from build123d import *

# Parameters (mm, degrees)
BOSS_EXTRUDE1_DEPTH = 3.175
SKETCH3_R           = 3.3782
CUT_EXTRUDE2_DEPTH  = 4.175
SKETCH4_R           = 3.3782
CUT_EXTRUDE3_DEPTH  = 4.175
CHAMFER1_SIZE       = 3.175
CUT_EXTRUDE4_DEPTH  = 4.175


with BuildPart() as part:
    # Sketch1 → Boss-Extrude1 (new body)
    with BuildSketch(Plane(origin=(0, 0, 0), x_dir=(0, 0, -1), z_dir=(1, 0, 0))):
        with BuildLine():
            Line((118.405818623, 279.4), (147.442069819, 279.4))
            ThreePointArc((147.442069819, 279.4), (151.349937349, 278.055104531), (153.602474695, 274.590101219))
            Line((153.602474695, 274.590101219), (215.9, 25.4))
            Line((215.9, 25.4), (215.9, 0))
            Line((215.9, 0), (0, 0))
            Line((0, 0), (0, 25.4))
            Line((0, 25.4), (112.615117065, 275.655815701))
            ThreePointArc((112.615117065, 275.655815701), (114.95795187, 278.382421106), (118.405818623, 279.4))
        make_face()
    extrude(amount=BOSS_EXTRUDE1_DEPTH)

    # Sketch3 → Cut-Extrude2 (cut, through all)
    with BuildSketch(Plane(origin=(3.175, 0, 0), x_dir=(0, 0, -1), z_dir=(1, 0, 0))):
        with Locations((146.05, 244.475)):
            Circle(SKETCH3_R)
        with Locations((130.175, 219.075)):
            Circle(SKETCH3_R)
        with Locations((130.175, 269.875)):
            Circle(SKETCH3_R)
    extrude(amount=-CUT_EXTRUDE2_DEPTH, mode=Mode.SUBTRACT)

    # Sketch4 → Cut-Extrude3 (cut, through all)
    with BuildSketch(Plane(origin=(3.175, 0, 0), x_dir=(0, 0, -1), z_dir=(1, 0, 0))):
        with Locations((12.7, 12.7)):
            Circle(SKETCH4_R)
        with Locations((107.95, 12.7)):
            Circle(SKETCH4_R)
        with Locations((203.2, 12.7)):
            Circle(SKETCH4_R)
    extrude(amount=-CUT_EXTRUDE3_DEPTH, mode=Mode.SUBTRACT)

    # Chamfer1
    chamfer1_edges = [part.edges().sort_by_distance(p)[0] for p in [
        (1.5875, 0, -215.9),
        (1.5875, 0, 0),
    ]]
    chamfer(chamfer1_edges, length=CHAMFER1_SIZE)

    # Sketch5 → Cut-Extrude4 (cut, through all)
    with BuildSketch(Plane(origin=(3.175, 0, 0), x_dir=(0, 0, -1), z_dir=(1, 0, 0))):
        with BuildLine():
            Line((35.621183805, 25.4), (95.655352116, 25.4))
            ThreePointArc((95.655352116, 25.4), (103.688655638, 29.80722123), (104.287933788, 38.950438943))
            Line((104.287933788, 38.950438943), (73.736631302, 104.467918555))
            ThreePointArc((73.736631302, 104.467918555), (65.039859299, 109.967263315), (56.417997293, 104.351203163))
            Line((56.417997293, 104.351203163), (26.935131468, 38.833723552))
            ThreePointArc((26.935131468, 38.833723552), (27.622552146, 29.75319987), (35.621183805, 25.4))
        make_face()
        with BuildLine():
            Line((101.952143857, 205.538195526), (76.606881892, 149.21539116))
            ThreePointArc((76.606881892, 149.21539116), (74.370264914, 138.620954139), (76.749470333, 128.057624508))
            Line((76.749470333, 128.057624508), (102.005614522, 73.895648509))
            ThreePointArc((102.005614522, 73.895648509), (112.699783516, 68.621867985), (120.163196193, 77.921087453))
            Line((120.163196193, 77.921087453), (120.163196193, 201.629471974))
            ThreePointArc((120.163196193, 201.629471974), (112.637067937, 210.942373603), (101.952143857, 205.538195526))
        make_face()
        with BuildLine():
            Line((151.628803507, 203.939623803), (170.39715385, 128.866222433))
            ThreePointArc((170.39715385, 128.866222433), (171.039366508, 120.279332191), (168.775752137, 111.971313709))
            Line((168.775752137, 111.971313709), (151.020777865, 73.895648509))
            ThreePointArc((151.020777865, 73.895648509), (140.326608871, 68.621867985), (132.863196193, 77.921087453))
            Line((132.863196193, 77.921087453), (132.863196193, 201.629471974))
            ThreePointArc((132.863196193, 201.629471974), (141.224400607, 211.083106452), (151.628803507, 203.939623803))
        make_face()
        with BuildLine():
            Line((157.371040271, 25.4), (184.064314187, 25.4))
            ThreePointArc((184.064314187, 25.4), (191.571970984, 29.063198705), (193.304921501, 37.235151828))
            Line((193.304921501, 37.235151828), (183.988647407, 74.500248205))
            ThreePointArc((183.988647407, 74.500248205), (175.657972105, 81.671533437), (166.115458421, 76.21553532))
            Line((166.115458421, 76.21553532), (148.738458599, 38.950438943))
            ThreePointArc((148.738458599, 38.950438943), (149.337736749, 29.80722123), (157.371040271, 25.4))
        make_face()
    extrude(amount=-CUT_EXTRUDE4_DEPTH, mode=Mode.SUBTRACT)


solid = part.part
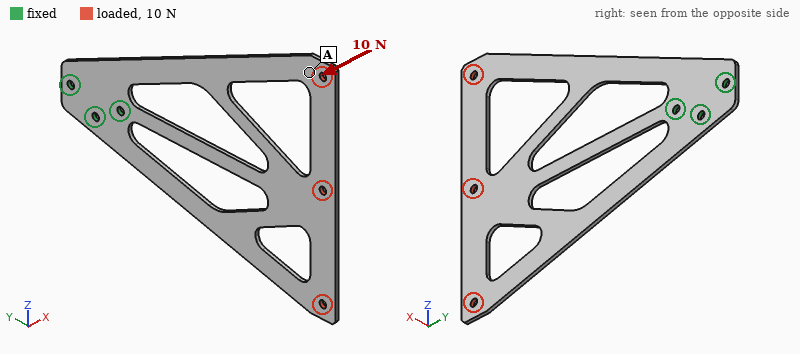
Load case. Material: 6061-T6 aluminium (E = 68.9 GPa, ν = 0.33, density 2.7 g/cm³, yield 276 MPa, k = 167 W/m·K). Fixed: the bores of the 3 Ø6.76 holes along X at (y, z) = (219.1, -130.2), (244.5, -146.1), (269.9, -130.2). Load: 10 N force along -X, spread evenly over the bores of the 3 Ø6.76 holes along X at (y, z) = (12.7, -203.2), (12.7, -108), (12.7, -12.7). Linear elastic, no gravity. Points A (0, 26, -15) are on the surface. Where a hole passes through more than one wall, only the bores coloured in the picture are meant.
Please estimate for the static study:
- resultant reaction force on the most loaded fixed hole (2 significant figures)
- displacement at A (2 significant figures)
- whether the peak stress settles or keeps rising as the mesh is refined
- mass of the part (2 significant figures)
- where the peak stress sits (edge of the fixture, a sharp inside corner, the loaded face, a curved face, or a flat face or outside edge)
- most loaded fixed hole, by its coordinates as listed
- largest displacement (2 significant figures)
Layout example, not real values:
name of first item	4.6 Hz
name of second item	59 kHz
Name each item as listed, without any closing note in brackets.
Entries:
resultant reaction force on the most loaded fixed hole	46 N
displacement at A	3.2 mm
whether the peak stress settles or keeps rising as the mesh is refined	keeps rising
mass of the part	200 g
where the peak stress sits	edge of the fixture
most loaded fixed hole, by its coordinates as listed	(219.1, -130.2)
largest displacement	3.8 mm
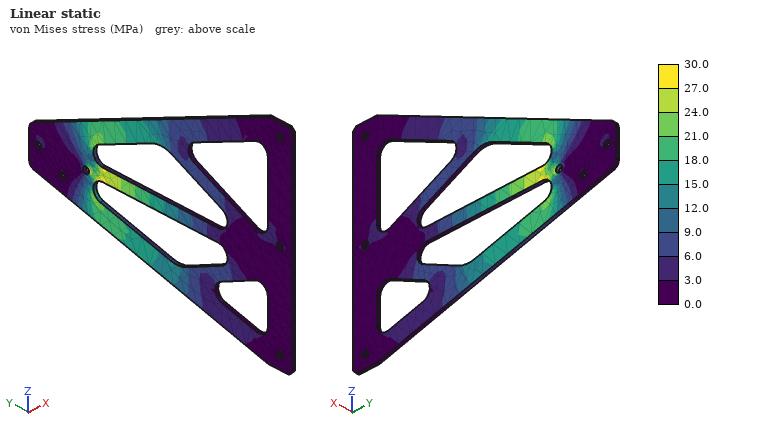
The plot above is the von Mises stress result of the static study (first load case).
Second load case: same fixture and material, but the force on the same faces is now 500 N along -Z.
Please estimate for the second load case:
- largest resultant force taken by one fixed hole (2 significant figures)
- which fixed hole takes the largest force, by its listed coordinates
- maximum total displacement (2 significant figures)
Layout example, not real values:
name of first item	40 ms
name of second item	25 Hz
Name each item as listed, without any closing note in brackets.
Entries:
largest resultant force taken by one fixed hole	2.6 kN
which fixed hole takes the largest force, by its listed coordinates	(219.1, -130.2)
maximum total displacement	1.2 mm
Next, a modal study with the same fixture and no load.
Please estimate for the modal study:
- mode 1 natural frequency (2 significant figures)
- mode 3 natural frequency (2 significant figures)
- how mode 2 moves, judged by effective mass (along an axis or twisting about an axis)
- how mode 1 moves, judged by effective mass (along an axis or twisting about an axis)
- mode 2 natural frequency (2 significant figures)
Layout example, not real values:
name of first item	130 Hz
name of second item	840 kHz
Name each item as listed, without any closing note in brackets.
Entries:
mode 1 natural frequency	32 Hz
mode 3 natural frequency	240 Hz
how mode 2 moves, judged by effective mass	twisting about Y
how mode 1 moves, judged by effective mass	along X
mode 2 natural frequency	75 Hz
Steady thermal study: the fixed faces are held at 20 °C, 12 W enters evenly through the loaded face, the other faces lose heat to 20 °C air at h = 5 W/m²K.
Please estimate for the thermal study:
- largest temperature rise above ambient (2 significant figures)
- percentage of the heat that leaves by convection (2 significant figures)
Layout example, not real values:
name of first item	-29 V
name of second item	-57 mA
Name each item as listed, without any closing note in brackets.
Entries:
largest temperature rise above ambient	49 K
percentage of the heat that leaves by convection	55 %
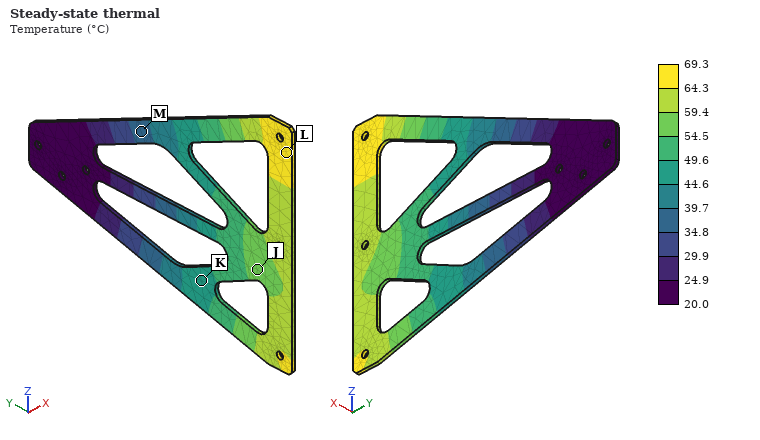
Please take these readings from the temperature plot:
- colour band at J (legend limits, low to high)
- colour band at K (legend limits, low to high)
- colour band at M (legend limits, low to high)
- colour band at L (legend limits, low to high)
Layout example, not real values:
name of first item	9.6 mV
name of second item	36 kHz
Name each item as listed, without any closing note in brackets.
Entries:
colour band at J	54.5 to 59.4 °C
colour band at K	44.6 to 49.6 °C
colour band at M	34.8 to 39.7 °C
colour band at L	64.3 to 69.3 °C
